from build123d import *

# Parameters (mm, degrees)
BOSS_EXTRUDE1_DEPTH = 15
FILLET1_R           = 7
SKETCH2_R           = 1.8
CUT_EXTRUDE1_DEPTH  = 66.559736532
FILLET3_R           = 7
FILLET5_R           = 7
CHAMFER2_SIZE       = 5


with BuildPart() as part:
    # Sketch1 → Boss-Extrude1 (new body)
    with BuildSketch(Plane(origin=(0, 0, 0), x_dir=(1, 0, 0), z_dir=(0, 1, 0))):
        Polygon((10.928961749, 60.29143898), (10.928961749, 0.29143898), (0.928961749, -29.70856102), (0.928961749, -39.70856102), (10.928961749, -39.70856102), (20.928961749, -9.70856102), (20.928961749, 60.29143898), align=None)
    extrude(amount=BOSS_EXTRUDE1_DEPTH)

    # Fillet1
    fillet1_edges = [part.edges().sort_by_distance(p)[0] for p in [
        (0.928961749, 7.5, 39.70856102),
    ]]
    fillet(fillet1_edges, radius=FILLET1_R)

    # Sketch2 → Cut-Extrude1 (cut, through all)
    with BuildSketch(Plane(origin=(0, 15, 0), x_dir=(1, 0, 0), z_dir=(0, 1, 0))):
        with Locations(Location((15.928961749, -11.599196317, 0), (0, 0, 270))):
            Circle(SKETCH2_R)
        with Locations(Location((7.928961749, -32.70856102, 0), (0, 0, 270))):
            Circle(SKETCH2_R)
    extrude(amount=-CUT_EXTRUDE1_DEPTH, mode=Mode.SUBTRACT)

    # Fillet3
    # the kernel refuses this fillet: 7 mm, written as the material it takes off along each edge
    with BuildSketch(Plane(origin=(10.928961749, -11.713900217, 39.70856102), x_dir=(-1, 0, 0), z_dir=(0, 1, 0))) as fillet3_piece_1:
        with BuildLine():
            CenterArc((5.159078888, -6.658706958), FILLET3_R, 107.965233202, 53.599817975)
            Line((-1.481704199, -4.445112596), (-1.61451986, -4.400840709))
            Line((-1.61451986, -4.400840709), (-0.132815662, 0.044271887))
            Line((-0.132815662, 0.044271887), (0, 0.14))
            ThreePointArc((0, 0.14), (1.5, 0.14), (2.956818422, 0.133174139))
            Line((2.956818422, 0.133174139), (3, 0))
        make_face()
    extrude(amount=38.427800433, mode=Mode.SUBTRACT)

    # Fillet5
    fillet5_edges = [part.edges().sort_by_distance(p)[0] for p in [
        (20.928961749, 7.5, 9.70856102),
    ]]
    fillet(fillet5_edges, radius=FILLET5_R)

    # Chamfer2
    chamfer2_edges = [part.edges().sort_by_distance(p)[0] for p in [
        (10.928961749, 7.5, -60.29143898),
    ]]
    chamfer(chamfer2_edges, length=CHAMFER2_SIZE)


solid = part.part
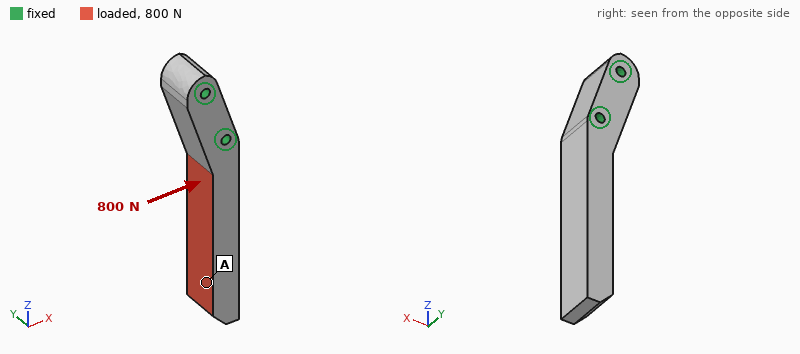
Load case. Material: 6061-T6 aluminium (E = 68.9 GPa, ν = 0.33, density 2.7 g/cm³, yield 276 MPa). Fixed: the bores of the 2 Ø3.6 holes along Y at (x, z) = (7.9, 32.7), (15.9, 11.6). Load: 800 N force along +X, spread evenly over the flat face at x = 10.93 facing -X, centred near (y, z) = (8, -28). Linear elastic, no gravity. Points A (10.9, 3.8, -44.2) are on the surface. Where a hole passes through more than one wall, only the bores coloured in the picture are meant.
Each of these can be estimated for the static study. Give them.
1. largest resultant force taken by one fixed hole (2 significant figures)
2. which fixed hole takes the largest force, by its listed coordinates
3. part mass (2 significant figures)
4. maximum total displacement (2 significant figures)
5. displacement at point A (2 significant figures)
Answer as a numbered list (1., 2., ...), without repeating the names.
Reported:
1. 1.8 kN
2. (15.9, 11.6)
3. 43 g
4. 0.43 mm
5. 0.30 mm
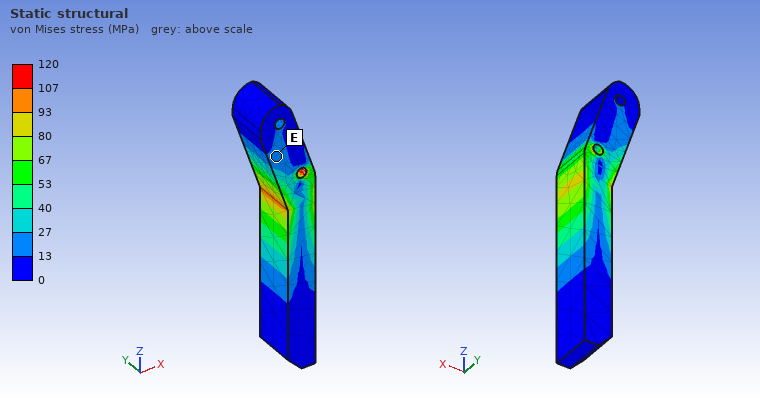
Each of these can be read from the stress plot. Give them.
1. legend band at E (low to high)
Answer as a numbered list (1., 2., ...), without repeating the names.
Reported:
1. 13 to 27 MPa
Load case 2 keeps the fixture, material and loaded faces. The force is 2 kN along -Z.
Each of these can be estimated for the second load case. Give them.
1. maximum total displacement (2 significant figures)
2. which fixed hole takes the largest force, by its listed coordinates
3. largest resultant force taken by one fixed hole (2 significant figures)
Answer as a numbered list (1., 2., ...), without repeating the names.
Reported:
1. 0.20 mm
2. (15.9, 11.6)
3. 1.5 kN
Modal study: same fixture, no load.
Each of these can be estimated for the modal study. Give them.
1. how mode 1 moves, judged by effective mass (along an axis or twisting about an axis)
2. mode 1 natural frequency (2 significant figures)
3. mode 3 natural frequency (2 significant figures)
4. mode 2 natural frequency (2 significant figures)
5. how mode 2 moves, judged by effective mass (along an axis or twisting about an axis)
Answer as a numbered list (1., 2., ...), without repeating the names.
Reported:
1. along X
2. 1700 Hz
3. 9500 Hz
4. 2400 Hz
5. along Y
